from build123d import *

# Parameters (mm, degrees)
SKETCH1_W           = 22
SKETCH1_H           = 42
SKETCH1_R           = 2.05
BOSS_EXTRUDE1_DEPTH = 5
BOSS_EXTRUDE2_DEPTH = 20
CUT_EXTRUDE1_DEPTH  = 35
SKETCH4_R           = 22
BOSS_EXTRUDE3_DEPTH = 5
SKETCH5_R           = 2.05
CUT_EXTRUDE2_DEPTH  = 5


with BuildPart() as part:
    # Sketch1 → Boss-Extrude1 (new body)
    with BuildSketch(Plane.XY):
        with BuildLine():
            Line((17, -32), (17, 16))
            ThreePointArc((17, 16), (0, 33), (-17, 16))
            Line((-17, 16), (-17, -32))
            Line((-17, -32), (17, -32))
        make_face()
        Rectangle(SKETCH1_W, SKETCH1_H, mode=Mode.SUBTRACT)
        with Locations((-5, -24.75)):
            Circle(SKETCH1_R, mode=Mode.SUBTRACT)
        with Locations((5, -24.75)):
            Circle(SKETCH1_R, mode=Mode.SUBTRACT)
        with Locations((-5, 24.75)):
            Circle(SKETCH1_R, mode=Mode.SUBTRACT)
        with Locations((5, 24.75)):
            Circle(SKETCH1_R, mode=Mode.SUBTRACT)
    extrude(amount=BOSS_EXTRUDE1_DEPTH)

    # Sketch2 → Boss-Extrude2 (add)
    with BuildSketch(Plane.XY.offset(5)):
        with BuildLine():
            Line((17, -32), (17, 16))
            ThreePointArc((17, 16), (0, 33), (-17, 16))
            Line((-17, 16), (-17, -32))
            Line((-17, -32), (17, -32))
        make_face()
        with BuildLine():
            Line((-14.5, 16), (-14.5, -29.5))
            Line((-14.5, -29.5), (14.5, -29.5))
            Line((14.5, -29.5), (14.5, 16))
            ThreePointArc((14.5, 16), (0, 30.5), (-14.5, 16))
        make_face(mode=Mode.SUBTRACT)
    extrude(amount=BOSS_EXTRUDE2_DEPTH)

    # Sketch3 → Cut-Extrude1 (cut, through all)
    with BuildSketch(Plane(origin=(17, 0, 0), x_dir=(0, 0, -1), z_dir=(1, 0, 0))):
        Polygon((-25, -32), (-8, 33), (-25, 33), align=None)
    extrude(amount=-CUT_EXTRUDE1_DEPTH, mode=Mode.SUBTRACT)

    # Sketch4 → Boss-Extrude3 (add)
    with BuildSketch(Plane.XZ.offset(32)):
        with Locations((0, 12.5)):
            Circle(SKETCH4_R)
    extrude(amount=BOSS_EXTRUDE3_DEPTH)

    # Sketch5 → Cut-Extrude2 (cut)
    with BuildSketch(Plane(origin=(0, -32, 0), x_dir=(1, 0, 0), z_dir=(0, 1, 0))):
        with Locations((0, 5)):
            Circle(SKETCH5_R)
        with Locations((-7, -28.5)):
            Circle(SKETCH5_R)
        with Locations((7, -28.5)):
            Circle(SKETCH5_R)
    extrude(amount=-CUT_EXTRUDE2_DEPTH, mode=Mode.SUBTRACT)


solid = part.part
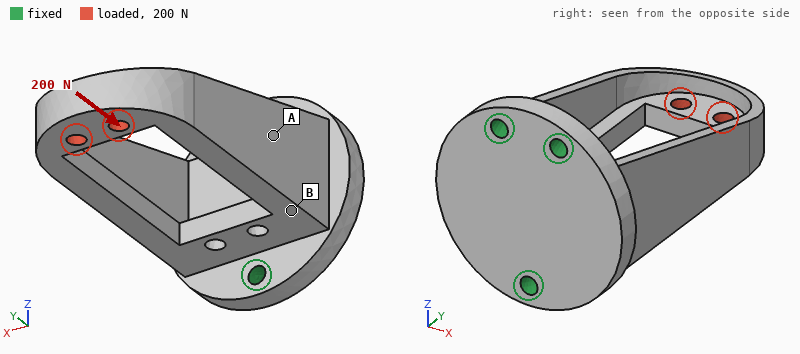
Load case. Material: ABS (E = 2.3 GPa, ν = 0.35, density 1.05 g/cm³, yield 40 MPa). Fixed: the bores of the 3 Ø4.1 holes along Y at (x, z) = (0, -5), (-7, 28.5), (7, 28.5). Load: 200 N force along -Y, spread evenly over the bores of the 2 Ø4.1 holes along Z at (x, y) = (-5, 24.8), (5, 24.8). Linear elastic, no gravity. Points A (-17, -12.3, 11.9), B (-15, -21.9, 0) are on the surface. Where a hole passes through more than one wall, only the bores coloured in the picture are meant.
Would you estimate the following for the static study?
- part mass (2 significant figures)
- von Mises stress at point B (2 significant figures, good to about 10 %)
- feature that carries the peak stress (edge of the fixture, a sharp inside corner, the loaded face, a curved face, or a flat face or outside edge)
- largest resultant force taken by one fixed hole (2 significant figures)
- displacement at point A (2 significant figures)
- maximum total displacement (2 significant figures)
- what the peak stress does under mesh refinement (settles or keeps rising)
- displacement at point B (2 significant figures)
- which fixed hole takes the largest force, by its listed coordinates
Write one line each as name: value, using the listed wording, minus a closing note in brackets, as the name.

part mass: 19 g
von Mises stress at point B: 3.5 MPa
feature that carries the peak stress: edge of the fixture
largest resultant force taken by one fixed hole: 170 N
displacement at point A: 0.090 mm
maximum total displacement: 0.35 mm
what the peak stress does under mesh refinement: keeps rising
displacement at point B: 0.071 mm
which fixed hole takes the largest force, by its listed coordinates: (0, -5)
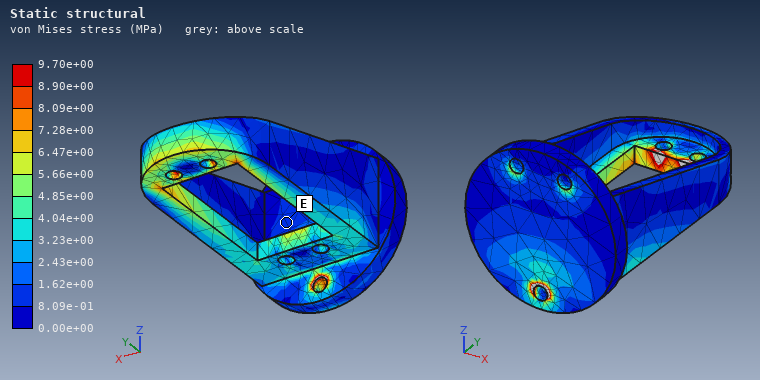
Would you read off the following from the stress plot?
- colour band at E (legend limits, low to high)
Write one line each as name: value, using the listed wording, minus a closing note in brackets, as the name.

colour band at E: 8.09e-01 to 1.62e+00 MPa
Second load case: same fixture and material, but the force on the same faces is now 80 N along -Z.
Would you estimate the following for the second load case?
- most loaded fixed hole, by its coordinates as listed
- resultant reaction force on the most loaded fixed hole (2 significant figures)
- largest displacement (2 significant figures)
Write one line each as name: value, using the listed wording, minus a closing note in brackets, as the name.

most loaded fixed hole, by its coordinates as listed: (0, -5)
resultant reaction force on the most loaded fixed hole: 170 N
largest displacement: 0.97 mm
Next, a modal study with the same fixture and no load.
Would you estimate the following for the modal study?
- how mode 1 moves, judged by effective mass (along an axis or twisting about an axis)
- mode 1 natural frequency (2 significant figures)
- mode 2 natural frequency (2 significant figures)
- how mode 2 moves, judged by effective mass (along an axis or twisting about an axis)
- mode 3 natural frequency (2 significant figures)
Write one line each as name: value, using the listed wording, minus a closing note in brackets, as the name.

how mode 1 moves, judged by effective mass: along X
mode 1 natural frequency: 460 Hz
mode 2 natural frequency: 950 Hz
how mode 2 moves, judged by effective mass: along Z
mode 3 natural frequency: 1600 Hz
